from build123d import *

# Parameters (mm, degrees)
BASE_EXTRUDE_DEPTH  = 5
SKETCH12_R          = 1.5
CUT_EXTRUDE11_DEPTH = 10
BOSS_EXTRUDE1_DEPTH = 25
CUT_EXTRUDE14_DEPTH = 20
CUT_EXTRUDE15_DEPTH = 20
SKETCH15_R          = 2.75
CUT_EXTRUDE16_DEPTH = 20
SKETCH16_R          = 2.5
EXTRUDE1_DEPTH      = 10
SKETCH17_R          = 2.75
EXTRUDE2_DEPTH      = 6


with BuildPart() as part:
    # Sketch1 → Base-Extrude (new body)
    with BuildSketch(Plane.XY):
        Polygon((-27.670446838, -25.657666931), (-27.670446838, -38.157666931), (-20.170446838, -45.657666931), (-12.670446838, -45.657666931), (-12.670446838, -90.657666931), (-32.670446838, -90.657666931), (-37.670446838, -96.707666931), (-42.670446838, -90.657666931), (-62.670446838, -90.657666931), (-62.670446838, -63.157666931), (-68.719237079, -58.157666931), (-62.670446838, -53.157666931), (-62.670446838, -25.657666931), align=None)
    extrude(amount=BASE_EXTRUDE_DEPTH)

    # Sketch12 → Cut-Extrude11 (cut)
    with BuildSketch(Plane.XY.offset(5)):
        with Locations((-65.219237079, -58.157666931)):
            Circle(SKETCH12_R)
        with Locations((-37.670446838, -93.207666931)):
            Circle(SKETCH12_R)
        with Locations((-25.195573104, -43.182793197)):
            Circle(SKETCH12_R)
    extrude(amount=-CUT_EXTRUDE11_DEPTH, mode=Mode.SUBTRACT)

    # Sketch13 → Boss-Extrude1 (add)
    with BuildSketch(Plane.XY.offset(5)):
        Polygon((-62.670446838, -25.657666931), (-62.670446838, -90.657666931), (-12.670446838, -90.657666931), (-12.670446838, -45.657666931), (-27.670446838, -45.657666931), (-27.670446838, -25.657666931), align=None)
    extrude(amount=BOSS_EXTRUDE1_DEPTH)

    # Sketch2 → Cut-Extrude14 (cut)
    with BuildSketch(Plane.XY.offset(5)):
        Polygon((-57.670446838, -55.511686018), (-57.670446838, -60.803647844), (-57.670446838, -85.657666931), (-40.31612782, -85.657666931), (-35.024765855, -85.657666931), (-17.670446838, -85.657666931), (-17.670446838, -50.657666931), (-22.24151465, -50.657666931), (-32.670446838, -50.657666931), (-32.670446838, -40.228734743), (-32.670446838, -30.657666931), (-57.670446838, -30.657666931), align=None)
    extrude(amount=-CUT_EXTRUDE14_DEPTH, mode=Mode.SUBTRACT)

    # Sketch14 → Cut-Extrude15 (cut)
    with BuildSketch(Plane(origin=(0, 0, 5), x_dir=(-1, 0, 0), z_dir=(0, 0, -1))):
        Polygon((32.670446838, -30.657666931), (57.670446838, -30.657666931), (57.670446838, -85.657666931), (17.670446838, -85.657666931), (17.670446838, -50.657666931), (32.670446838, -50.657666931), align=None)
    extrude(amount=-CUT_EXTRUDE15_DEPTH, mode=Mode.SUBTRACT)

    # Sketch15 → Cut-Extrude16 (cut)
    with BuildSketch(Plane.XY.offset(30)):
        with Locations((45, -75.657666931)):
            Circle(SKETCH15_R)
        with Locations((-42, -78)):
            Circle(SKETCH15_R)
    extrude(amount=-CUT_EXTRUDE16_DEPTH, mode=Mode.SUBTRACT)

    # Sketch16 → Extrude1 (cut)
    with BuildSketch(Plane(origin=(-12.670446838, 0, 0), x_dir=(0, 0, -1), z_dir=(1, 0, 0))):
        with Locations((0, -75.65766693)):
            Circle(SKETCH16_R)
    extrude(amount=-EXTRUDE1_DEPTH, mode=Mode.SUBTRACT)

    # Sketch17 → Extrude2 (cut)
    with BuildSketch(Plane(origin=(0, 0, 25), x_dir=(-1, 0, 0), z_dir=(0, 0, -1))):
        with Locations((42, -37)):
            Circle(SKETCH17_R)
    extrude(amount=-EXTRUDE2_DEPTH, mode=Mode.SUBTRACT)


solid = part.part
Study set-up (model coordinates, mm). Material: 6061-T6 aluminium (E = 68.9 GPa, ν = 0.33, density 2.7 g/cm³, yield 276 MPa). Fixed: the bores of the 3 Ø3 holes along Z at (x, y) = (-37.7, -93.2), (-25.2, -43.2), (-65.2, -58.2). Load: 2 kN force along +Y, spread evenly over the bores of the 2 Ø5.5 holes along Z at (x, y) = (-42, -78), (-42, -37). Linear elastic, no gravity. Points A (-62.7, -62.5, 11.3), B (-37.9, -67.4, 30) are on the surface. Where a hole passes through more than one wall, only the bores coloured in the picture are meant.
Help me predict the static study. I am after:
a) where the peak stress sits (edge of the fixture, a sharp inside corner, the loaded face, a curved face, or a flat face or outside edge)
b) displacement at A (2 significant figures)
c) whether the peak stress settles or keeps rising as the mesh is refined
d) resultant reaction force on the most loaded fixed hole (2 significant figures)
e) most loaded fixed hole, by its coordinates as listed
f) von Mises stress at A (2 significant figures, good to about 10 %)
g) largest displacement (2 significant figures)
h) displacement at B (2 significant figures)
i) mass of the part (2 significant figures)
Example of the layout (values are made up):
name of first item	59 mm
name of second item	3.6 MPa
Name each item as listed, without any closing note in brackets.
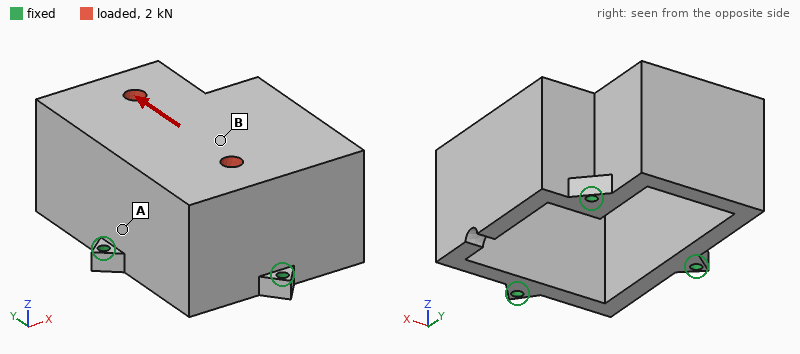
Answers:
where the peak stress sits	edge of the fixture
displacement at A	11 µm
whether the peak stress settles or keeps rising as the mesh is refined	keeps rising
resultant reaction force on the most loaded fixed hole	1.2 kN
most loaded fixed hole, by its coordinates as listed	(-37.7, -93.2)
von Mises stress at A	15 MPa
largest displacement	36 µm
displacement at B	25 µm
mass of the part	110 g
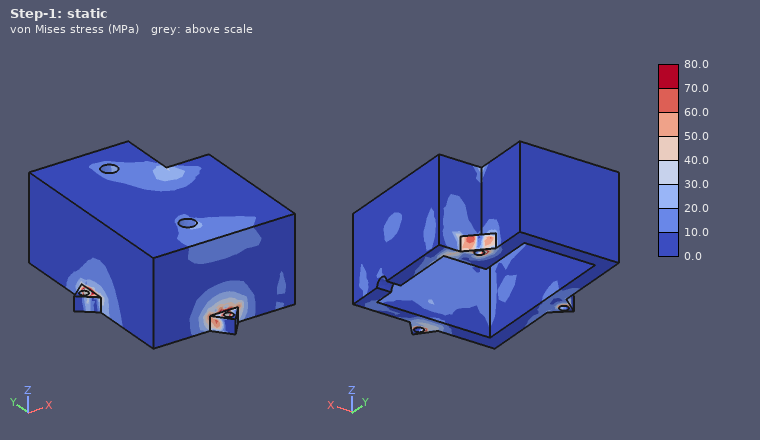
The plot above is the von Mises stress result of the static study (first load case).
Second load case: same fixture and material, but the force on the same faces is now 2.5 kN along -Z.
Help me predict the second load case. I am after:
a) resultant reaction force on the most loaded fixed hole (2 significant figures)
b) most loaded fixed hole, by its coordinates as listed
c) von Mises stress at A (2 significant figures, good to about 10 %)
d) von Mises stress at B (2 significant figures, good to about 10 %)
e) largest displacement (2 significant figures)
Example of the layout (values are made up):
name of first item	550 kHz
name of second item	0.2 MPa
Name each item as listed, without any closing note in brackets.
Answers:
resultant reaction force on the most loaded fixed hole	1.1 kN
most loaded fixed hole, by its coordinates as listed	(-25.2, -43.2)
von Mises stress at A	13 MPa
von Mises stress at B	17 MPa
largest displacement	25 µm
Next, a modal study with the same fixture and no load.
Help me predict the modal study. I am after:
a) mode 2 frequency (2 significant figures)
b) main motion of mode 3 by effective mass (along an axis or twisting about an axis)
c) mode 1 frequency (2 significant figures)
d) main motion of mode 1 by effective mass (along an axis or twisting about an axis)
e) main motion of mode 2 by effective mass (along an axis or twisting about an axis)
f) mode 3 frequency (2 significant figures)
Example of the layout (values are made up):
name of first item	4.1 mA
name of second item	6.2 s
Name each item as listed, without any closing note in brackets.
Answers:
mode 2 frequency	4900 Hz
main motion of mode 3 by effective mass	twisting about Z
mode 1 frequency	4200 Hz
main motion of mode 1 by effective mass	along X
main motion of mode 2 by effective mass	along Y
mode 3 frequency	6800 Hz
